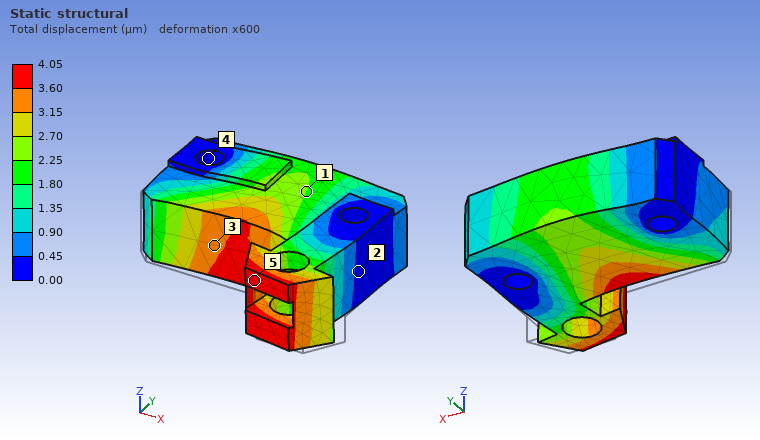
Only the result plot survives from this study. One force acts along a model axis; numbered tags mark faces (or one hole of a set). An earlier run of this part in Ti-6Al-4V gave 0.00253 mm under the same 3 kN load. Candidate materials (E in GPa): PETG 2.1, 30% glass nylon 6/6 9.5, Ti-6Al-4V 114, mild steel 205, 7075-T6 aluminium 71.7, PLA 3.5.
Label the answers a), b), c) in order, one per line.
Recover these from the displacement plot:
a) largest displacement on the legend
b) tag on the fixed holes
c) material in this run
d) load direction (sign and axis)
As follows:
a) 4.05 µm
b) 4
c) 7075-T6 aluminium
d) +Y
